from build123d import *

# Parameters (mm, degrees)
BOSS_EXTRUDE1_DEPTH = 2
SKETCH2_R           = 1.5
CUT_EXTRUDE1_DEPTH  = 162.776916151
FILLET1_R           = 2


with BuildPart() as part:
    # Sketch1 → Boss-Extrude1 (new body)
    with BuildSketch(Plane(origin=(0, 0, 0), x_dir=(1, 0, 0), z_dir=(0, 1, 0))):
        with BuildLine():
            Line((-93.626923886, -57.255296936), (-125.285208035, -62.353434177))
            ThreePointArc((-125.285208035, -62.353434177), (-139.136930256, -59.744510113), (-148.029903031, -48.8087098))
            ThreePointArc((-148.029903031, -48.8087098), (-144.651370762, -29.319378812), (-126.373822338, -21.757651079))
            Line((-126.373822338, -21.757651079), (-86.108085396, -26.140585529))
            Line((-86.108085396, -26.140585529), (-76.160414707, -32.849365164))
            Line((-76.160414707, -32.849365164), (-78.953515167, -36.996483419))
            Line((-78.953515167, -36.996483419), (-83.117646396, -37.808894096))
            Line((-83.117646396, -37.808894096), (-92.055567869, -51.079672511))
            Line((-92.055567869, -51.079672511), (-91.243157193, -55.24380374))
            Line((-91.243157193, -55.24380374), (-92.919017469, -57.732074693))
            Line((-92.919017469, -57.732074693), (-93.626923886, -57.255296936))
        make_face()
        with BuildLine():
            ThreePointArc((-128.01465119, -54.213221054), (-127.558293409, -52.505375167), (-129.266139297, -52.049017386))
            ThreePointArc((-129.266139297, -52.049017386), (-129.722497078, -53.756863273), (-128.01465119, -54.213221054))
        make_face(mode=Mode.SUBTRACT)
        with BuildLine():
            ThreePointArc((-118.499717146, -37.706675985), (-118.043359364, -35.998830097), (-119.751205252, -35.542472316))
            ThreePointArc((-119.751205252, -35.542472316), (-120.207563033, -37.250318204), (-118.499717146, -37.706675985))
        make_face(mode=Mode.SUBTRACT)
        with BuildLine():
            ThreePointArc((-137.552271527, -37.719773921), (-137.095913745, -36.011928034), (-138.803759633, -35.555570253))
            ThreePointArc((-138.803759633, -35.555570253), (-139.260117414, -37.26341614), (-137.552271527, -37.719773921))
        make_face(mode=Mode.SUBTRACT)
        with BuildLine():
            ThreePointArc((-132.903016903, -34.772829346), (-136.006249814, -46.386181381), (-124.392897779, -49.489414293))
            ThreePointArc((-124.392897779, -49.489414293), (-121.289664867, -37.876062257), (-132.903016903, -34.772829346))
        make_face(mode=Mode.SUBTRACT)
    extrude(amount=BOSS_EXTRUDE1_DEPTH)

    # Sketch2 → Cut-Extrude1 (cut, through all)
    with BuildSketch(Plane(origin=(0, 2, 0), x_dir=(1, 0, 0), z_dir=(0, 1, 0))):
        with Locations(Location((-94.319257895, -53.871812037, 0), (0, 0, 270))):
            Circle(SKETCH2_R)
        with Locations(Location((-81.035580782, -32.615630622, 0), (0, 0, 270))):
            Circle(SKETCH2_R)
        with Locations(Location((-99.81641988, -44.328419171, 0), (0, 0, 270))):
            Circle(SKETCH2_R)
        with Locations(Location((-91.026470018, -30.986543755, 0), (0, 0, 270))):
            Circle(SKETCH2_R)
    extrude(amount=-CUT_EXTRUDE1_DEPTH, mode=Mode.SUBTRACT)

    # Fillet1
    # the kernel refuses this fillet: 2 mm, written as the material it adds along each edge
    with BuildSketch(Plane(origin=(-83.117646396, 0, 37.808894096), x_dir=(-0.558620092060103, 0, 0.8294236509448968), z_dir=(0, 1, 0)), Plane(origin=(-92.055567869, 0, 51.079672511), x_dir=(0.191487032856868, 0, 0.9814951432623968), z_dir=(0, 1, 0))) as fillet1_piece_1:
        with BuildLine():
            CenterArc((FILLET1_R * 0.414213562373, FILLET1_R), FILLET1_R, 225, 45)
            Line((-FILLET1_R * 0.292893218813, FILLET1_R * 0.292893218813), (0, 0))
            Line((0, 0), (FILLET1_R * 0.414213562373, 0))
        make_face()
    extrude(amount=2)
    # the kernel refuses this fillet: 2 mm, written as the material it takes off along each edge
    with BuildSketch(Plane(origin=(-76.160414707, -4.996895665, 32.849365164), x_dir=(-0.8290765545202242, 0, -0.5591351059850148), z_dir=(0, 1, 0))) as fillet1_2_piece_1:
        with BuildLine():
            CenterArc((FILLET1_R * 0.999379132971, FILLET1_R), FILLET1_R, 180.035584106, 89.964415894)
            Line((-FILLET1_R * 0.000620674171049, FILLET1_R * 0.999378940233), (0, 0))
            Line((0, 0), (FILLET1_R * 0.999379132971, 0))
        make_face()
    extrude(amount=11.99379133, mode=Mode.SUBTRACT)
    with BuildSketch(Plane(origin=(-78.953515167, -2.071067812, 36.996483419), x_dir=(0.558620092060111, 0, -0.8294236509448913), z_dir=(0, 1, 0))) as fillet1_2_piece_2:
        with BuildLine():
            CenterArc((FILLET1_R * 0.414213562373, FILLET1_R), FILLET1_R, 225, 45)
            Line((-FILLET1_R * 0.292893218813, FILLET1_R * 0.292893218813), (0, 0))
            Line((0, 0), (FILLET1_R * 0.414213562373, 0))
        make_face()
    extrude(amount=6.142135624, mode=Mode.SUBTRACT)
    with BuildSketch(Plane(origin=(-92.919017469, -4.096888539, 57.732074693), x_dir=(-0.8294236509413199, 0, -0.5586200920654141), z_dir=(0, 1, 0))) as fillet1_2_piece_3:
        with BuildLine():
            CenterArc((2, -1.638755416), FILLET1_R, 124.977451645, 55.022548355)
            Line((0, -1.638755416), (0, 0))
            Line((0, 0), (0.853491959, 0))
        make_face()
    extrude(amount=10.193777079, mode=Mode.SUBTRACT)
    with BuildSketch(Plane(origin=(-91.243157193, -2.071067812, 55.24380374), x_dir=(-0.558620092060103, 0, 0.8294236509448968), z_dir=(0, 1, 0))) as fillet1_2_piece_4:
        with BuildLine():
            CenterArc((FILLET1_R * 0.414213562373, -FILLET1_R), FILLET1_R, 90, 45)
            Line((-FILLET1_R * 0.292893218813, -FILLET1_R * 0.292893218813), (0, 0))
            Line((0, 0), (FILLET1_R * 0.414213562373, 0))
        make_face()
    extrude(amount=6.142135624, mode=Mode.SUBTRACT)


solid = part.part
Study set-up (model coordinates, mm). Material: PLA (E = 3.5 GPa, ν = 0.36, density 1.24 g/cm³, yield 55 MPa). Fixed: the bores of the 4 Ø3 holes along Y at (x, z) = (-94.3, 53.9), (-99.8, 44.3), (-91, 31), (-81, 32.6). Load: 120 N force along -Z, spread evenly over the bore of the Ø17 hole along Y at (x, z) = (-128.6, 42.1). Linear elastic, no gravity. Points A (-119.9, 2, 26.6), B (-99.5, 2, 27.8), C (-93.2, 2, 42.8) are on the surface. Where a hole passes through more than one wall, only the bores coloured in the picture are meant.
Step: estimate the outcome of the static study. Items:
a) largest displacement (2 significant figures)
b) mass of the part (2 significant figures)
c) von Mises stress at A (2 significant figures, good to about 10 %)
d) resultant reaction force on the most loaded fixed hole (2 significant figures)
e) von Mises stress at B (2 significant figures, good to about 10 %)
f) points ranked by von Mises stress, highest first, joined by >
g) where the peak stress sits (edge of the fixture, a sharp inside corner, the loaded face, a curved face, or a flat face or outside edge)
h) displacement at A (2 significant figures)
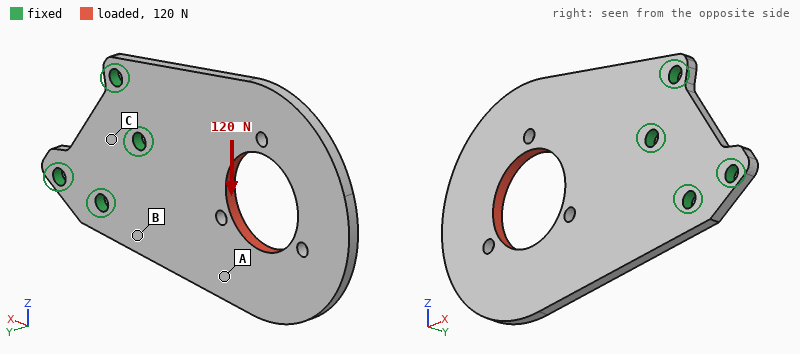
0.24 mm
4.8 g
3.2 MPa
130 N
6.9 MPa
B > A > C
edge of the fixture
0.11 mm
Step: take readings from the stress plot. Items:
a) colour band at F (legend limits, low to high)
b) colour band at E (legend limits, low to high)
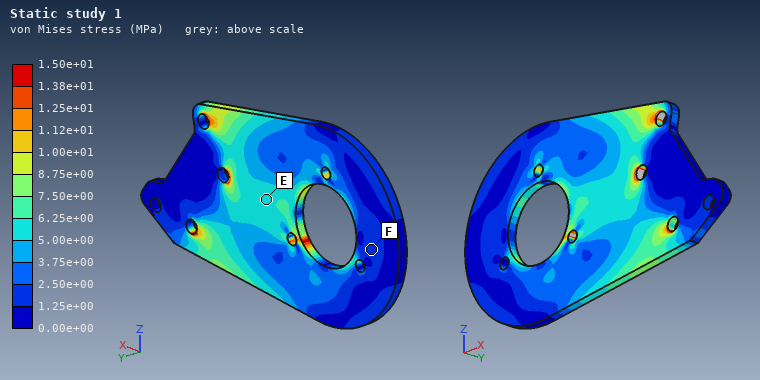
1.25e+00 to 2.50e+00 MPa
5.00e+00 to 6.25e+00 MPa
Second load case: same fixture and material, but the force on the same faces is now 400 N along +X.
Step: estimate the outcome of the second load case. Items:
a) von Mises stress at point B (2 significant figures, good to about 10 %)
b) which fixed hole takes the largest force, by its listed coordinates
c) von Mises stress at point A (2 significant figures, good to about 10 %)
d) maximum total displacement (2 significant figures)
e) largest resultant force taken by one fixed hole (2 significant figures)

6.0 MPa
(-99.8, 44.3)
4.9 MPa
0.11 mm
160 N
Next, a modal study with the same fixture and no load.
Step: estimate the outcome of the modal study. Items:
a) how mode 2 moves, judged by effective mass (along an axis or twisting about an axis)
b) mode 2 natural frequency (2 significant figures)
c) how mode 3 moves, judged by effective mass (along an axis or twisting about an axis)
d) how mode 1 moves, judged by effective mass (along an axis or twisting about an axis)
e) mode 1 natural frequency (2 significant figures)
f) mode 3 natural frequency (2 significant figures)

twisting about X
590 Hz
along Y
along Y
250 Hz
1200 Hz
